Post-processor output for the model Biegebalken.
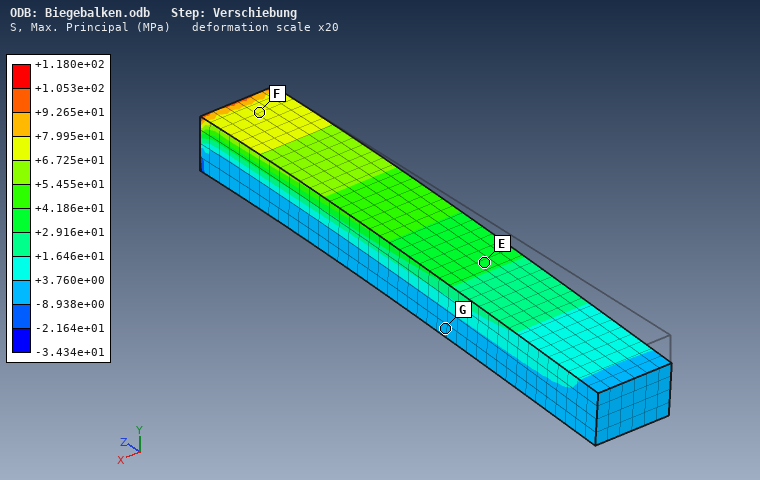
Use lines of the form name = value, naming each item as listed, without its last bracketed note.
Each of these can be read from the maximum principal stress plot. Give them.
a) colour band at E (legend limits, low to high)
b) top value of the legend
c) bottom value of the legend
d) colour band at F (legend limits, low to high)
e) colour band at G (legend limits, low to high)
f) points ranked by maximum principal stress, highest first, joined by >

colour band at E = +2.916e+01 to +4.186e+01 MPa
top value of the legend = +1.180e+02 MPa
bottom value of the legend = -3.434e+01 MPa
colour band at F = +6.725e+01 to +7.995e+01 MPa
colour band at G = -8.938e+00 to +3.760e+00 MPa
points ranked by maximum principal stress, highest first, joined by > = F > E > G
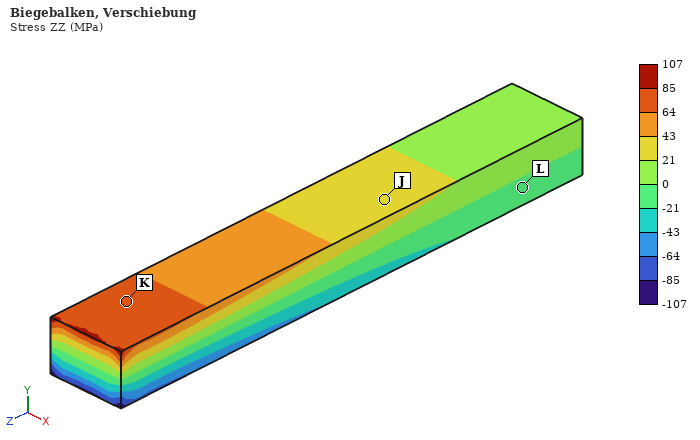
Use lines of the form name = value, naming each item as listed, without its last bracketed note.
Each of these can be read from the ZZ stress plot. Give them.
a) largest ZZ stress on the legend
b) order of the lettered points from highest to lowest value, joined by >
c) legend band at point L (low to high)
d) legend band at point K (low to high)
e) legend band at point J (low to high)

largest ZZ stress on the legend = 107 MPa
order of the lettered points from highest to lowest value, joined by > = K > J > L
legend band at point L = -21 to 0 MPa
legend band at point K = 64 to 85 MPa
legend band at point J = 21 to 43 MPa
